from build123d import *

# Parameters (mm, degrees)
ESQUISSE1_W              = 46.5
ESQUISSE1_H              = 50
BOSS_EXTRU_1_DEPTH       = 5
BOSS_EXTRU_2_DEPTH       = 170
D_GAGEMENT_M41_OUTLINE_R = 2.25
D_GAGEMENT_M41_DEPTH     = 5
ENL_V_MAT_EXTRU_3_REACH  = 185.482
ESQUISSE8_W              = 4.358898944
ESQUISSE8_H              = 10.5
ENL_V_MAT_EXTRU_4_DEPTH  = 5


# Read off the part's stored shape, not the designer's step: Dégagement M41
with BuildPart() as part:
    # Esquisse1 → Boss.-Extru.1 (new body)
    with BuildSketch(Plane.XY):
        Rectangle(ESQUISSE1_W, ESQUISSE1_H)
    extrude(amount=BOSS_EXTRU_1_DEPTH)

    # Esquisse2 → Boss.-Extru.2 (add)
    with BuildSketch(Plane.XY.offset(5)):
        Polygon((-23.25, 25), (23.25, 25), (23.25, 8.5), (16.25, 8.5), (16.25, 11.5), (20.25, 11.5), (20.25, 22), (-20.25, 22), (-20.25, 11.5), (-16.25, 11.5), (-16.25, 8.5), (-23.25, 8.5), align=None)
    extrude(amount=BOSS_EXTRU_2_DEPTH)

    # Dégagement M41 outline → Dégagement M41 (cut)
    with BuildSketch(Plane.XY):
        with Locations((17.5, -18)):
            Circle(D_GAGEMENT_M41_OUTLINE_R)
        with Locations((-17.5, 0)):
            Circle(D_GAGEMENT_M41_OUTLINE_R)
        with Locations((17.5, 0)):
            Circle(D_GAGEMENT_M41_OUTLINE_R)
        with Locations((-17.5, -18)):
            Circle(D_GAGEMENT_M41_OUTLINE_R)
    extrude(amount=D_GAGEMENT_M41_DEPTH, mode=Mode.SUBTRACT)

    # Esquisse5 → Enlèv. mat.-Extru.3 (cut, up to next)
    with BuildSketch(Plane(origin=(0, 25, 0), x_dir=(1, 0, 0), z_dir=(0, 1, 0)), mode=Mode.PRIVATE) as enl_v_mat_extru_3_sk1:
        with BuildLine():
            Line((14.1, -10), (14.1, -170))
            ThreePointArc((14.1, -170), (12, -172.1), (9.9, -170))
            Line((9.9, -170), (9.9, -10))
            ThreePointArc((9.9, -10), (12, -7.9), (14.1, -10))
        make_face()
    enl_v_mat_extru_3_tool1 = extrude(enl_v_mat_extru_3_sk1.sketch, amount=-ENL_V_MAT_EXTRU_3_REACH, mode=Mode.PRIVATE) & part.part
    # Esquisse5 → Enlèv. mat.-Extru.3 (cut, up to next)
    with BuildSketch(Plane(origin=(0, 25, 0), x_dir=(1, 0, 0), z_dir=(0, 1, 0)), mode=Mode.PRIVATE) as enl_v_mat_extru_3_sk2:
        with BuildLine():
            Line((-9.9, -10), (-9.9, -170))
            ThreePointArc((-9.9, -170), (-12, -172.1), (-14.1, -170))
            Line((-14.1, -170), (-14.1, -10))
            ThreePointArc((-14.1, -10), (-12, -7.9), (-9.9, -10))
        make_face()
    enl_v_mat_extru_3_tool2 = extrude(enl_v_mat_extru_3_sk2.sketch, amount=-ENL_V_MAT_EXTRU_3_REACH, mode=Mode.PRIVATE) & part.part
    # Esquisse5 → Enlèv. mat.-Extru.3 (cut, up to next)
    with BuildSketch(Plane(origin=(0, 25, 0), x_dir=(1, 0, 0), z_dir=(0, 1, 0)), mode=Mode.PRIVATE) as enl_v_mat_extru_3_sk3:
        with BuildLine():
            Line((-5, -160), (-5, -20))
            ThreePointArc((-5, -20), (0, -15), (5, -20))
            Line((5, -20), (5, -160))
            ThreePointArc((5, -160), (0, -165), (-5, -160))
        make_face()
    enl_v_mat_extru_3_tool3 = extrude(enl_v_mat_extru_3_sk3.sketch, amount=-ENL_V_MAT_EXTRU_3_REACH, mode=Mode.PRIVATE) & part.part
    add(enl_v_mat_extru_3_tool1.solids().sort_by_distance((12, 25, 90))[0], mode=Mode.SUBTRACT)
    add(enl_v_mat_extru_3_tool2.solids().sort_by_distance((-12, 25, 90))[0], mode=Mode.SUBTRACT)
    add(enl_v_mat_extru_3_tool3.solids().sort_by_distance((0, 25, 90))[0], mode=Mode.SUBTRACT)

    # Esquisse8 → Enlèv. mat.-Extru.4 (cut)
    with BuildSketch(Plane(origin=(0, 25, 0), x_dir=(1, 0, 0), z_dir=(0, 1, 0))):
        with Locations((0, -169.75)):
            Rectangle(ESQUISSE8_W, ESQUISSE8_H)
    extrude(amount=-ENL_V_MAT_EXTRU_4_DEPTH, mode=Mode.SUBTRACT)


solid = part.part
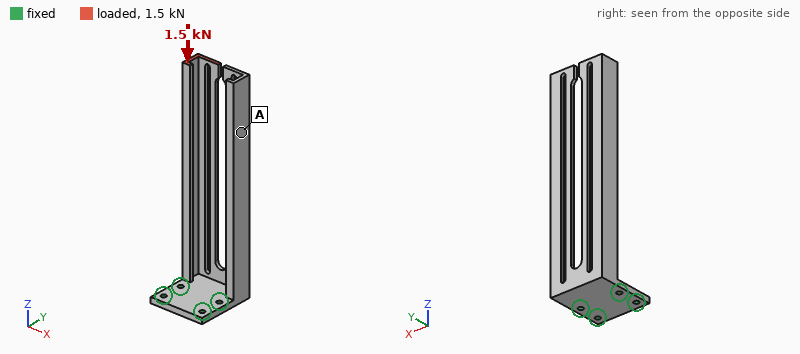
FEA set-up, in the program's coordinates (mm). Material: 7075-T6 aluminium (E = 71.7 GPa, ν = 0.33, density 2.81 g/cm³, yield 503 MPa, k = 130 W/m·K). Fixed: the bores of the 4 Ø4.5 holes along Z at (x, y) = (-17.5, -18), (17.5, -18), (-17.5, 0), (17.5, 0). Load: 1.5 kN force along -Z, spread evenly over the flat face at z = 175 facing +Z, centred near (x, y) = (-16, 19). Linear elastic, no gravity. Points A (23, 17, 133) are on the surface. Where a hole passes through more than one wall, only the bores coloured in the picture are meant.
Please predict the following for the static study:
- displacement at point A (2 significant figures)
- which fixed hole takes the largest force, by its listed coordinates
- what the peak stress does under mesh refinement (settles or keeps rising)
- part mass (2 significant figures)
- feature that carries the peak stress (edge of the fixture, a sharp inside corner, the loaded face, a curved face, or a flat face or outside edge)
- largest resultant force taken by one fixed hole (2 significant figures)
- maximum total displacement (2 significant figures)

0.69 mm
(-17.5, 0)
keeps rising
120 g
edge of the fixture
1.7 kN
2.0 mm
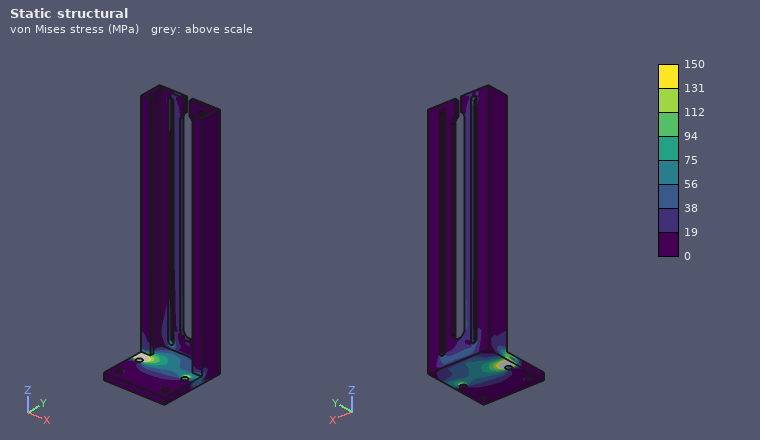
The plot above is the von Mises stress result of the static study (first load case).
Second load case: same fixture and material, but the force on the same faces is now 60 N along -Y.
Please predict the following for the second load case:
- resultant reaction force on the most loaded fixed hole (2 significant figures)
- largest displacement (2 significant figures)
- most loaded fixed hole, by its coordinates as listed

120 N
2.0 mm
(-17.5, 0)
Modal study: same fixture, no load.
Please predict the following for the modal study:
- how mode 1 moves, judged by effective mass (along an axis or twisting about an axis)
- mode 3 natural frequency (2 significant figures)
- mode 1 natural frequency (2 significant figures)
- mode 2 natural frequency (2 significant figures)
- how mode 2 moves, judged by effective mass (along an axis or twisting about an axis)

along X
240 Hz
200 Hz
220 Hz
along Y
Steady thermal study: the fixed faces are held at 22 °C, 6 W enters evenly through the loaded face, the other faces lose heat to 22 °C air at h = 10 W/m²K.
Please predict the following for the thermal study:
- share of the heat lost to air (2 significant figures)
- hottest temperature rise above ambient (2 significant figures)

56 %
57 K
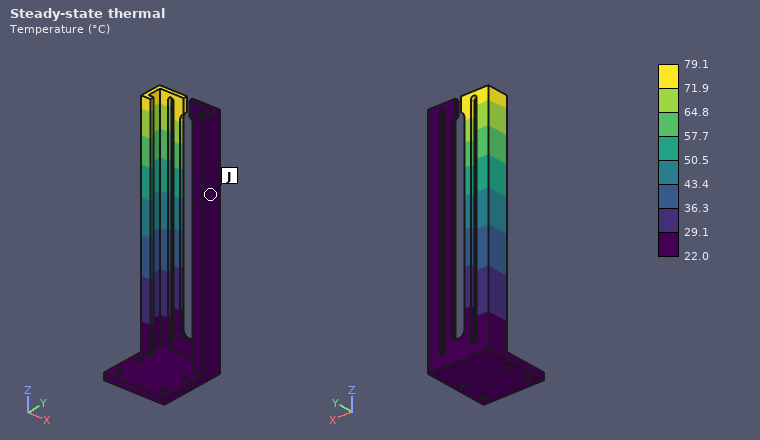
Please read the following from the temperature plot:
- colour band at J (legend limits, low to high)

22.0 to 29.1 °C
